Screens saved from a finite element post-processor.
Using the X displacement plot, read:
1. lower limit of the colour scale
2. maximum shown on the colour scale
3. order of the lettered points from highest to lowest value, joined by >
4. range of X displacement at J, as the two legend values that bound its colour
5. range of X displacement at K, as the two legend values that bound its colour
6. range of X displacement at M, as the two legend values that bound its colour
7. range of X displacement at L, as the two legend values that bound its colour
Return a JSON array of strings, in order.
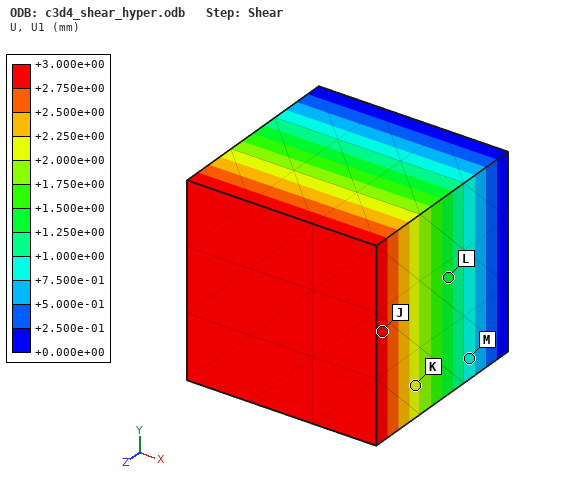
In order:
["+0.000e+00 mm", "+3.000e+00 mm", "J > K > L > M", "+2.750e+00 to +3.000e+00 mm", "+2.000e+00 to +2.250e+00 mm", "+7.500e-01 to +1.000e+00 mm", "+1.250e+00 to +1.500e+00 mm"]
